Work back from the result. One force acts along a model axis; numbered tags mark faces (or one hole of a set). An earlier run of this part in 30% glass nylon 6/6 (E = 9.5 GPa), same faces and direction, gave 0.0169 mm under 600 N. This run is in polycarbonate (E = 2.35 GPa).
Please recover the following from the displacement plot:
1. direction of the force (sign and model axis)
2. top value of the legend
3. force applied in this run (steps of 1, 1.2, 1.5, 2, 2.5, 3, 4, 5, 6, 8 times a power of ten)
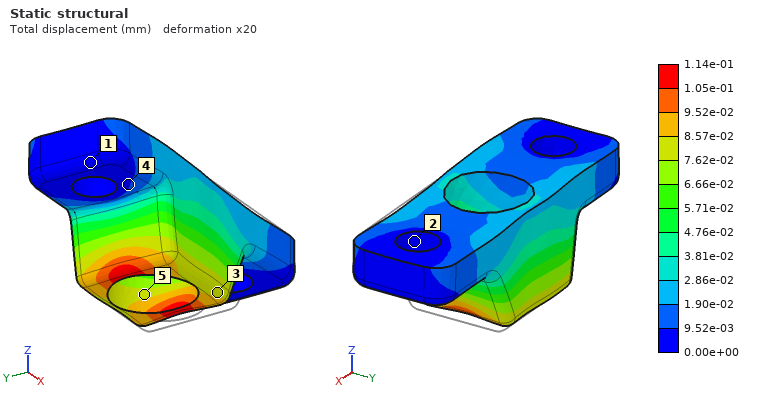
-X
1.14e-01 mm
1 kN
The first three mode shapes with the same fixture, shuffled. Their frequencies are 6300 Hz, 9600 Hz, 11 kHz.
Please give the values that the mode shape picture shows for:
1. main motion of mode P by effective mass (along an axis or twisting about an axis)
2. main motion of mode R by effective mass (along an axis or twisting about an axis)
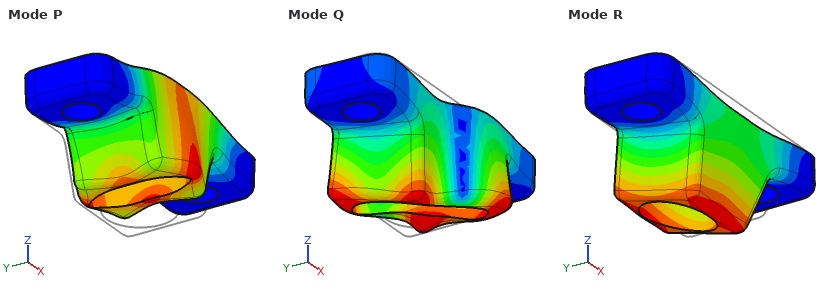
along Z
along Y
